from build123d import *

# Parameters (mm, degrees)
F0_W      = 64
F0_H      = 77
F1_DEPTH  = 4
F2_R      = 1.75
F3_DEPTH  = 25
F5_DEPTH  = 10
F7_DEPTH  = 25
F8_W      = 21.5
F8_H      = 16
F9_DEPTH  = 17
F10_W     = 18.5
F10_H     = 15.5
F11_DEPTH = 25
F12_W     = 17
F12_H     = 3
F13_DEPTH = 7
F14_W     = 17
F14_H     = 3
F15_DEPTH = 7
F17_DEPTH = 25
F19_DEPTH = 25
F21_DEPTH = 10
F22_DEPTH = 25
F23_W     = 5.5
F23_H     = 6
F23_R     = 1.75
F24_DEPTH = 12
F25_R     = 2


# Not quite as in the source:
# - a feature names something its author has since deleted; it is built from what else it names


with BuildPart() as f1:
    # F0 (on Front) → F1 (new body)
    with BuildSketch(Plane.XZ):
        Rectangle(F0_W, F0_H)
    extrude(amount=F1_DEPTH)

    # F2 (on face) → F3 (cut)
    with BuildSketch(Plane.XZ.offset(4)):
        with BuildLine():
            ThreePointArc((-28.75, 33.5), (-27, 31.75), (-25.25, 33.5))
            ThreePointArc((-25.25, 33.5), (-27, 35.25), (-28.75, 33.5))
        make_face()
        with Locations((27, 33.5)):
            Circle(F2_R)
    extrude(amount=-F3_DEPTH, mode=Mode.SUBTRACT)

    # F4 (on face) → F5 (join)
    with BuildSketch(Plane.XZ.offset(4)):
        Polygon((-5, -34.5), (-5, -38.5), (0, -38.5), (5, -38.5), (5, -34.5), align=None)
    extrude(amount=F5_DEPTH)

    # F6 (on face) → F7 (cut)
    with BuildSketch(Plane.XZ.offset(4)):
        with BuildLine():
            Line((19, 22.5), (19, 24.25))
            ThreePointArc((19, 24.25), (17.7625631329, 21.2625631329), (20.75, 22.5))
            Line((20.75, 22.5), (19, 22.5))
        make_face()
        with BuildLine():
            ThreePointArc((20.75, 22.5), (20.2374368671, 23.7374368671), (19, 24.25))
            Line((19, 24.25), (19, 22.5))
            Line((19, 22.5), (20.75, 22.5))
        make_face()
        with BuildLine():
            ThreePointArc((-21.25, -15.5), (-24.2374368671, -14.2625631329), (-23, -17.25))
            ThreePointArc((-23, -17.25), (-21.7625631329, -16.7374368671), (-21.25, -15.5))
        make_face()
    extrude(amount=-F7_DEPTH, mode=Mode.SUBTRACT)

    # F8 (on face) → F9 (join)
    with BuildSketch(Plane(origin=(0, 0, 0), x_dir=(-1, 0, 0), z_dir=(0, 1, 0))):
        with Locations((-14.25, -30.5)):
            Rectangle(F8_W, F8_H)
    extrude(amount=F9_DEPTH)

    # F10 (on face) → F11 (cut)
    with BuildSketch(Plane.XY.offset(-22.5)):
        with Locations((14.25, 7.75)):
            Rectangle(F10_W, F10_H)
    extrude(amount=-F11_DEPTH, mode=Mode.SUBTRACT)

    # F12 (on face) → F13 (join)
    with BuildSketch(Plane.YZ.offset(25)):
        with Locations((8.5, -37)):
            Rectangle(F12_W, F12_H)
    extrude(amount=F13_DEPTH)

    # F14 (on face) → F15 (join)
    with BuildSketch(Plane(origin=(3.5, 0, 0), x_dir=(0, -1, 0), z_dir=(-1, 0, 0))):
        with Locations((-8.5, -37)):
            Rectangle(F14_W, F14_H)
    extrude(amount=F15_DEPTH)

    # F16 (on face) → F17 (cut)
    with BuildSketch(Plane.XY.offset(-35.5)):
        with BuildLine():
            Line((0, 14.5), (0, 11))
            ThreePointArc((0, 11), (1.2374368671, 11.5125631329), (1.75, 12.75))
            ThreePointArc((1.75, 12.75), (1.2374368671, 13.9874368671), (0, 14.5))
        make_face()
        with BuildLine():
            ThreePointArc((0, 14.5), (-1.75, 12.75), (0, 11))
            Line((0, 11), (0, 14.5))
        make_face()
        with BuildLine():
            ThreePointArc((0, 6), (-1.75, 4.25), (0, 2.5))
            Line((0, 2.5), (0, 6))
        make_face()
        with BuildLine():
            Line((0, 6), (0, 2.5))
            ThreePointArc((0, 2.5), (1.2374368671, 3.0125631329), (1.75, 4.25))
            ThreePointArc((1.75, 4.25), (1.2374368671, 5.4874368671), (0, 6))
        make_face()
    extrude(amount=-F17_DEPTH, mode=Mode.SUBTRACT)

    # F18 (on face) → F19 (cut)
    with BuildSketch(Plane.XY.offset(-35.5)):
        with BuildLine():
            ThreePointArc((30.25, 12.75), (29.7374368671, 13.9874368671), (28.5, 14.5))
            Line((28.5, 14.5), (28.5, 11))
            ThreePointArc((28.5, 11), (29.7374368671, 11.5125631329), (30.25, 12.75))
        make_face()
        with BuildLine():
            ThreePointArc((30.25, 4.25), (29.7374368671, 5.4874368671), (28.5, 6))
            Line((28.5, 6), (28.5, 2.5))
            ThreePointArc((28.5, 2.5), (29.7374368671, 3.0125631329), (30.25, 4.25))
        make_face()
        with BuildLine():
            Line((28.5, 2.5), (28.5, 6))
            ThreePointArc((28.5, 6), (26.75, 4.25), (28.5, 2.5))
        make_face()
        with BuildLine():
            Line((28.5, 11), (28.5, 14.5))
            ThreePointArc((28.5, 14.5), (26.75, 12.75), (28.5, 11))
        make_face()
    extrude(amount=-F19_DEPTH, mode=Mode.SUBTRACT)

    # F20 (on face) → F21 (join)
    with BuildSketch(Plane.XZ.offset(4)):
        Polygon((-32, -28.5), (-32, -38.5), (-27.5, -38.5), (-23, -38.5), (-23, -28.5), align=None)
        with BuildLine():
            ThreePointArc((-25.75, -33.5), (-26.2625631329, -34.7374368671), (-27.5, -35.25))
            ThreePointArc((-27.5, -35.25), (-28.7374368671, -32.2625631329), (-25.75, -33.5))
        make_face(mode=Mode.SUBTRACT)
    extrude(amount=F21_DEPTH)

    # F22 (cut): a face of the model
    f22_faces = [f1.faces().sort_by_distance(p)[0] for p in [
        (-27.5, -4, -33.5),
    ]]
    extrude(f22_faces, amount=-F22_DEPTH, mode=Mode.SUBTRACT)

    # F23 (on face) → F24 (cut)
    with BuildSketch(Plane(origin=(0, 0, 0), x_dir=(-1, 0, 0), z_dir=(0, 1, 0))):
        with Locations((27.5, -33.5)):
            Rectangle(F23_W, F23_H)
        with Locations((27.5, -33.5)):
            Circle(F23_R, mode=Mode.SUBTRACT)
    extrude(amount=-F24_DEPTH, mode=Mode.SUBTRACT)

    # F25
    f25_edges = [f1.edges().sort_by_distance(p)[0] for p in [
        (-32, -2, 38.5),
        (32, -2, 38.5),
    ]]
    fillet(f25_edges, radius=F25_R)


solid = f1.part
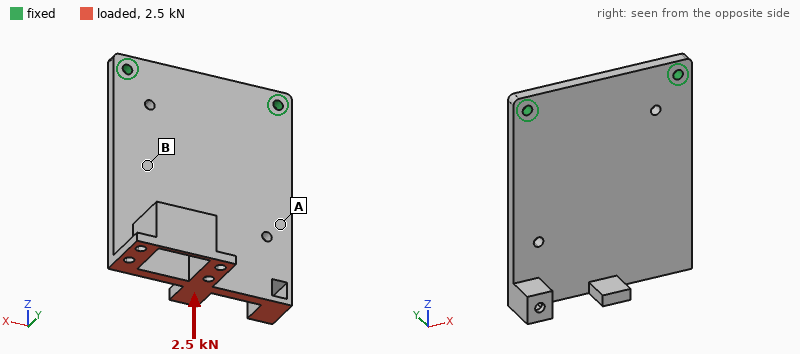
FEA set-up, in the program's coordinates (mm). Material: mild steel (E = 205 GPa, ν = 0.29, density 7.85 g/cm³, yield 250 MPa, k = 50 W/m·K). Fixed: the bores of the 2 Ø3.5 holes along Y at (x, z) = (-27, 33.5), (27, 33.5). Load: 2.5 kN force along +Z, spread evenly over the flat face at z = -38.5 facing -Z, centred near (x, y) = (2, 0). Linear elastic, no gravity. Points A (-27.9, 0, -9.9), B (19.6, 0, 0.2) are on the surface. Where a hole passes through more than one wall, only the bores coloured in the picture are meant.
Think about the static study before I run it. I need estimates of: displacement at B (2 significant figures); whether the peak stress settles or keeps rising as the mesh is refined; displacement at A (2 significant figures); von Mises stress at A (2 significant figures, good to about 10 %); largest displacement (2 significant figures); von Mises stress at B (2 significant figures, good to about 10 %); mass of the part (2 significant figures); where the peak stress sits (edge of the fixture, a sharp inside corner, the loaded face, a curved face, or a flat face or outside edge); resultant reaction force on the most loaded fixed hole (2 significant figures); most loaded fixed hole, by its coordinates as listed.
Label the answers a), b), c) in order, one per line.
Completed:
a) 0.076 mm
b) keeps rising
c) 0.10 mm
d) 30 MPa
e) 0.37 mm
f) 52 MPa
g) 180 g
h) edge of the fixture
i) 1.4 kN
j) (27, 33.5)
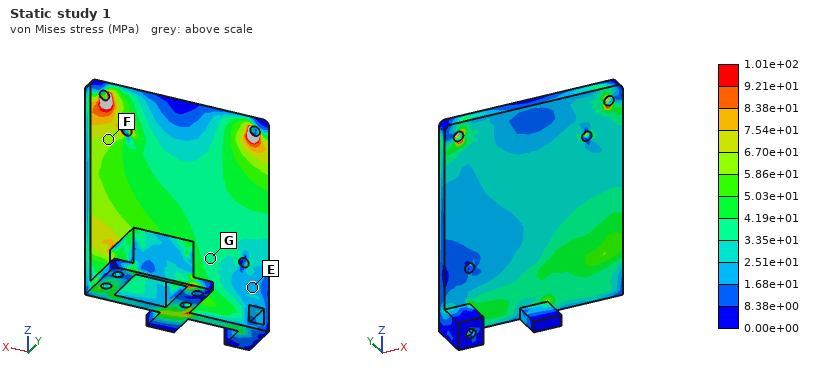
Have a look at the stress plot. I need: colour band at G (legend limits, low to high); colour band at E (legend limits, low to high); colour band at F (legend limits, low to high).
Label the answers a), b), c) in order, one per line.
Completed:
a) 3.35e+01 to 4.19e+01 MPa
b) 1.68e+01 to 2.51e+01 MPa
c) 5.86e+01 to 6.70e+01 MPa
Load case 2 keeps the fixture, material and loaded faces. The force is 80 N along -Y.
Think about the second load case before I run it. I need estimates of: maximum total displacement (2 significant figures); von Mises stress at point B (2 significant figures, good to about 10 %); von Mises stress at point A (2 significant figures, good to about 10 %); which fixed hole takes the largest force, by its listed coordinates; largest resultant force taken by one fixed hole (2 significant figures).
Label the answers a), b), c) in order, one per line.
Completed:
a) 0.20 mm
b) 19 MPa
c) 14 MPa
d) (27, 33.5)
e) 43 N
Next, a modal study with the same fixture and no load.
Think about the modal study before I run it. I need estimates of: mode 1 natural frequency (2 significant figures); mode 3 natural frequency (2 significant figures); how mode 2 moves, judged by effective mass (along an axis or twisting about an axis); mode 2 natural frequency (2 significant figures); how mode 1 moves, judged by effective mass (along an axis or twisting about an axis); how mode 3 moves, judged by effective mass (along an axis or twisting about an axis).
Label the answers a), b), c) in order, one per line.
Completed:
a) 440 Hz
b) 2800 Hz
c) twisting about Z
d) 1400 Hz
e) along Y
f) along Y
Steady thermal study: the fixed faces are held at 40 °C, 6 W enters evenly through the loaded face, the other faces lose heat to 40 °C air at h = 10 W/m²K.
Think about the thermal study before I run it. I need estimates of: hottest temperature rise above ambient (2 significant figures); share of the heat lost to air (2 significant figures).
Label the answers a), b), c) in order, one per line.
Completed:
a) 32 K
b) 38 %
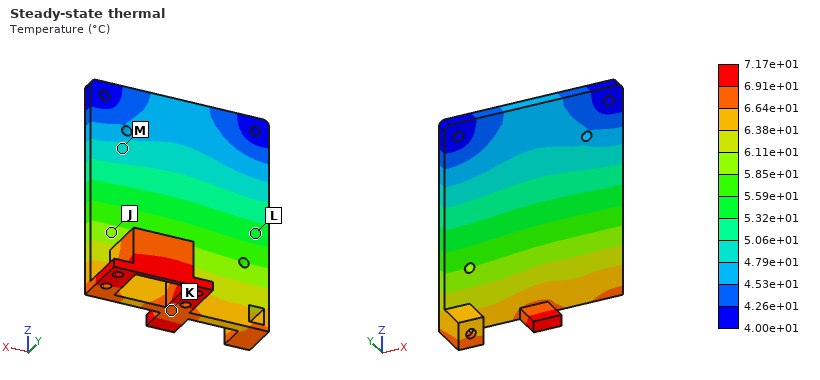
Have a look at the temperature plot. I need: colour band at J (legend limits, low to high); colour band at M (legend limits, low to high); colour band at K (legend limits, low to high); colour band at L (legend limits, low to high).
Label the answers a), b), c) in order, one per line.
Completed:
a) 5.85e+01 to 6.11e+01 °C
b) 4.79e+01 to 5.06e+01 °C
c) 6.64e+01 to 6.91e+01 °C
d) 5.32e+01 to 5.59e+01 °C
